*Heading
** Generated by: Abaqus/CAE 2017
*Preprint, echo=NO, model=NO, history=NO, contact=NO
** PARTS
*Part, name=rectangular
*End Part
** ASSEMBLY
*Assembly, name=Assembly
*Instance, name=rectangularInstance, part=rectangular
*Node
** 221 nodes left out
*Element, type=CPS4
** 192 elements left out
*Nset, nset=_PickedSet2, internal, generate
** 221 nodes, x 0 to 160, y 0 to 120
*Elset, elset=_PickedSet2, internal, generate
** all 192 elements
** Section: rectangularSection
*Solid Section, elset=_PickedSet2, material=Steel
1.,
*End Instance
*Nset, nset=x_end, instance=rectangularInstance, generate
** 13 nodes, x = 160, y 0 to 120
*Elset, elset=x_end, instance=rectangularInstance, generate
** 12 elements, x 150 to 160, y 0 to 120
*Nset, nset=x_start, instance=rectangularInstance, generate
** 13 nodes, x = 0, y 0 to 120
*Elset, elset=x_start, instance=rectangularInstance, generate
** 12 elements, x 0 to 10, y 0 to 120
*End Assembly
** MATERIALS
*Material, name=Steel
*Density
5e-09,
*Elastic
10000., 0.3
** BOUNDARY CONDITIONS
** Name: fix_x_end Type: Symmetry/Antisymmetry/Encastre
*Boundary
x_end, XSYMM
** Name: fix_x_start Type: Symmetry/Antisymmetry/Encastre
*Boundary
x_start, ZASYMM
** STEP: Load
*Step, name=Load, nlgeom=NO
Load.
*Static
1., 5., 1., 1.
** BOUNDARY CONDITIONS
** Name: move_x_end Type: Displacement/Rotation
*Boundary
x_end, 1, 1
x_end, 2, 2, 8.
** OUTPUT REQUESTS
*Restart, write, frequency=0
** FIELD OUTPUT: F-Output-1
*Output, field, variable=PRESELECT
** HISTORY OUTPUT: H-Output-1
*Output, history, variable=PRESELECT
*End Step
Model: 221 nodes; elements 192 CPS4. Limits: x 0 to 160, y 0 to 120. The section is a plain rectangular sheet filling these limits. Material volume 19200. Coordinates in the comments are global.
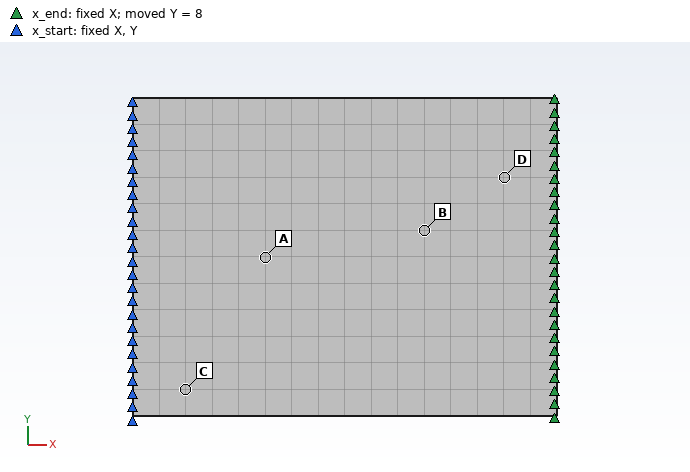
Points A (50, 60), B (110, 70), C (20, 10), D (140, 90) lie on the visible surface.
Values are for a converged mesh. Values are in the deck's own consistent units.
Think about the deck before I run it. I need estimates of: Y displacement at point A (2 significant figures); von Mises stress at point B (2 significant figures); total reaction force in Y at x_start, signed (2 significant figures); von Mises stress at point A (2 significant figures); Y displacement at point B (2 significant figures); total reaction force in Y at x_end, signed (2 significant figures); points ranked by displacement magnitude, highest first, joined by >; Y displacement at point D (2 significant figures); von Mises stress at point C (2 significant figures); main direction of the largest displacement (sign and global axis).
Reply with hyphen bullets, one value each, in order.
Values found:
- 2.2
- 260
- -13000
- 270
- 5.8
- 13000
- D > B > A > C
- 7.3
- 310
- +Y
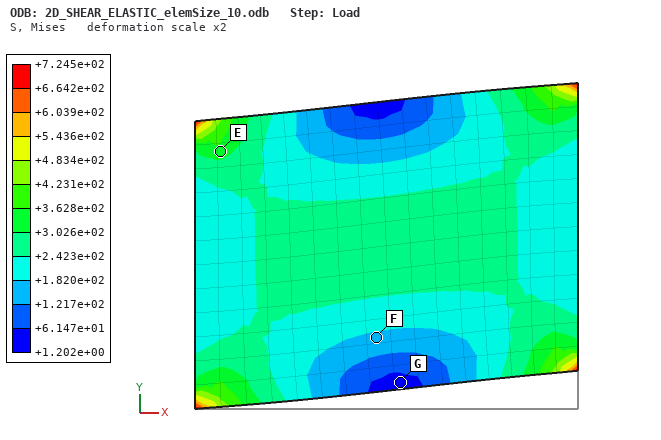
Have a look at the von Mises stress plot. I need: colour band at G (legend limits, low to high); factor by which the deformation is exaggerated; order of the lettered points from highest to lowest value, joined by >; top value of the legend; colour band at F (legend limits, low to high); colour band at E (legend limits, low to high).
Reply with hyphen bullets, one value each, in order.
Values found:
- +1.202e+00 to +6.147e+01
- 2
- E > F > G
- +7.245e+02
- +1.217e+02 to +1.820e+02
- +3.026e+02 to +3.628e+02
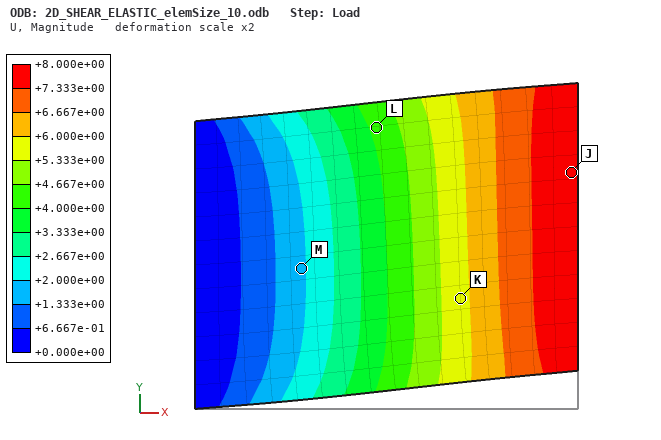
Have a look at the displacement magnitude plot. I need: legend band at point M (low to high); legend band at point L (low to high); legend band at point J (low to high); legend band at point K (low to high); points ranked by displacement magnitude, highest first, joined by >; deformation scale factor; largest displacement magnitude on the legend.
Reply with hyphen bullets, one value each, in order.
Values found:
- +1.333e+00 to +2.000e+00
- +4.000e+00 to +4.667e+00
- +7.333e+00 to +8.000e+00
- +5.333e+00 to +6.000e+00
- J > K > L > M
- 2
- +8.000e+00
